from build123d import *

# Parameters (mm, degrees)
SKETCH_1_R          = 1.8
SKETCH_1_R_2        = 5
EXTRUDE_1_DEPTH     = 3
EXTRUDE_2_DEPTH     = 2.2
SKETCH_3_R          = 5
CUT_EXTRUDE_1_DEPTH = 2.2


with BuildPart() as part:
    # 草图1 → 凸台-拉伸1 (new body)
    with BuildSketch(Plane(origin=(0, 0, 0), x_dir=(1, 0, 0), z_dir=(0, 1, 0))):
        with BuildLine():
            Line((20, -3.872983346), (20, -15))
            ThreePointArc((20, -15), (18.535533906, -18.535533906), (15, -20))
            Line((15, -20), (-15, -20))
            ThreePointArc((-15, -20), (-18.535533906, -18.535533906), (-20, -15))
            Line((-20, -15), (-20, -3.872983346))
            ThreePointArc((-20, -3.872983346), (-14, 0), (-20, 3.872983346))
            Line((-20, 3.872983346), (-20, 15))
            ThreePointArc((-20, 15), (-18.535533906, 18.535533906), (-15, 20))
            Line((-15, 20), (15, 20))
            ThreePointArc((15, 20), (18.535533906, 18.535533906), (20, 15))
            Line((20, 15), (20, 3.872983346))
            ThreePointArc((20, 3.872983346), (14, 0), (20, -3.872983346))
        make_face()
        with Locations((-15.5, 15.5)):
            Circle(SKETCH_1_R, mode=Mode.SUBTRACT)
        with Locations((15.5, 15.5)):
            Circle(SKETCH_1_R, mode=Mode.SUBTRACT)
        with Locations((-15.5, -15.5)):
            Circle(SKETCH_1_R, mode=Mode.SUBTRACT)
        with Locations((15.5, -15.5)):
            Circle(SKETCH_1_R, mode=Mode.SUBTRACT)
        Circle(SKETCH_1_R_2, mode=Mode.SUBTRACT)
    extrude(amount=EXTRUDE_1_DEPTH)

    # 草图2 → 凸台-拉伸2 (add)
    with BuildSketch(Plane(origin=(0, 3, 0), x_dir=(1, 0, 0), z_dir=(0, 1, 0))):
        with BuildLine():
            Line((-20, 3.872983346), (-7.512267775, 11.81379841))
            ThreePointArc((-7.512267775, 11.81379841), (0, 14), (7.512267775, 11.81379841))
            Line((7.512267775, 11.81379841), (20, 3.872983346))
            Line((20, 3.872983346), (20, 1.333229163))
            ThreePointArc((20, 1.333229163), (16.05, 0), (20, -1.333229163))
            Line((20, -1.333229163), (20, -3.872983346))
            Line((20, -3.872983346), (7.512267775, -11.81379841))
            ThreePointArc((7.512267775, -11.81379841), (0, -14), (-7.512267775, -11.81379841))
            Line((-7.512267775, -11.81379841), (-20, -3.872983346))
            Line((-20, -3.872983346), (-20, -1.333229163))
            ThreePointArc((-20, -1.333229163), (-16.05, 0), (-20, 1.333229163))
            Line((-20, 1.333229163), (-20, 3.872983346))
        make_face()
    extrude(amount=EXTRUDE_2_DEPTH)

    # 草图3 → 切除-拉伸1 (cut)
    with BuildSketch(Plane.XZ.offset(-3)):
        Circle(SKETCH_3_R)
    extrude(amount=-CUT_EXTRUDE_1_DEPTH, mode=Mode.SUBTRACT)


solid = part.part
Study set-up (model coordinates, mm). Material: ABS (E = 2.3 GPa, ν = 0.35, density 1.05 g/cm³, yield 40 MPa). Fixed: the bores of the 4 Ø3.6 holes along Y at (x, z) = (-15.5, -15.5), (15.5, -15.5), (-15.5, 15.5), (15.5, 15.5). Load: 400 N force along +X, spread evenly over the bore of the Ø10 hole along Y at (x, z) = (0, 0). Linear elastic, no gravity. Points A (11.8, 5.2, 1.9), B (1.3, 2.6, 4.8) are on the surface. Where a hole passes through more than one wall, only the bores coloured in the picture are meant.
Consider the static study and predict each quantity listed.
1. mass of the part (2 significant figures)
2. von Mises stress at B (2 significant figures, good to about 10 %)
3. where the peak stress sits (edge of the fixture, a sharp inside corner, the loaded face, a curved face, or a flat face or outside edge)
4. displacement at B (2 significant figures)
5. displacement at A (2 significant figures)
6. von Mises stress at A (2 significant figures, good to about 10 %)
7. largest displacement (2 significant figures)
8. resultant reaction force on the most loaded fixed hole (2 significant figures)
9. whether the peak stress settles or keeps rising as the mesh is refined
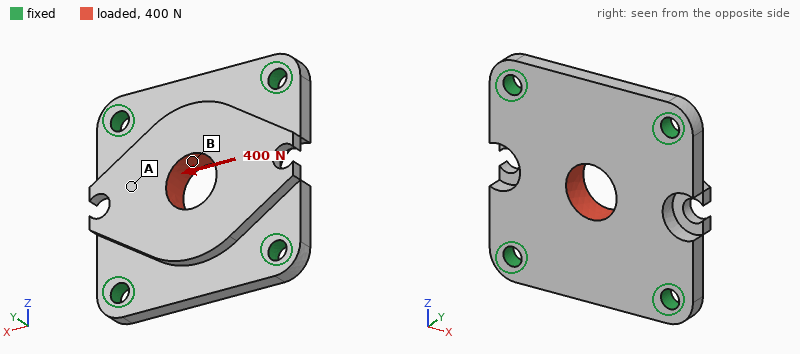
5.9 g
4.3 MPa
edge of the fixture
29 µm
28 µm
1.3 MPa
33 µm
120 N
keeps rising
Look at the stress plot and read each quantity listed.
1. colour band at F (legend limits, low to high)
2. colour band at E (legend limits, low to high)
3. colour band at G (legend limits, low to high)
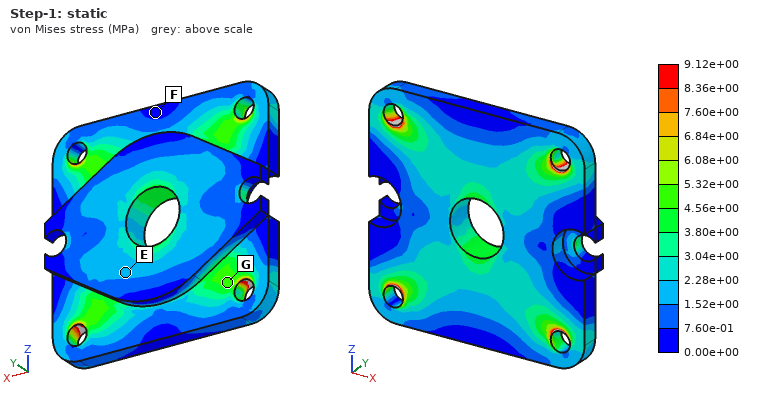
0.00e+00 to 7.60e-01 MPa
1.52e+00 to 2.28e+00 MPa
4.56e+00 to 5.32e+00 MPa
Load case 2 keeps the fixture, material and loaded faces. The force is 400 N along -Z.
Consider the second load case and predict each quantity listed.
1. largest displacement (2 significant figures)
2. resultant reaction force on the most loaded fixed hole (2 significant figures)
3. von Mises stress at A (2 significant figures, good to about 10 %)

33 µm
110 N
1.3 MPa
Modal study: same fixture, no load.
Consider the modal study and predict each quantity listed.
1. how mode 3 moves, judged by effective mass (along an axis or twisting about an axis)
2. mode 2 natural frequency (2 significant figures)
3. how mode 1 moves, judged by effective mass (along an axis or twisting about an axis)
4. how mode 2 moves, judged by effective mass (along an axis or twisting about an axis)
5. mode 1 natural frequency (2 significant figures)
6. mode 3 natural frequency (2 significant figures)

twisting about Z
5800 Hz
along Y
twisting about X
3900 Hz
6100 Hz
